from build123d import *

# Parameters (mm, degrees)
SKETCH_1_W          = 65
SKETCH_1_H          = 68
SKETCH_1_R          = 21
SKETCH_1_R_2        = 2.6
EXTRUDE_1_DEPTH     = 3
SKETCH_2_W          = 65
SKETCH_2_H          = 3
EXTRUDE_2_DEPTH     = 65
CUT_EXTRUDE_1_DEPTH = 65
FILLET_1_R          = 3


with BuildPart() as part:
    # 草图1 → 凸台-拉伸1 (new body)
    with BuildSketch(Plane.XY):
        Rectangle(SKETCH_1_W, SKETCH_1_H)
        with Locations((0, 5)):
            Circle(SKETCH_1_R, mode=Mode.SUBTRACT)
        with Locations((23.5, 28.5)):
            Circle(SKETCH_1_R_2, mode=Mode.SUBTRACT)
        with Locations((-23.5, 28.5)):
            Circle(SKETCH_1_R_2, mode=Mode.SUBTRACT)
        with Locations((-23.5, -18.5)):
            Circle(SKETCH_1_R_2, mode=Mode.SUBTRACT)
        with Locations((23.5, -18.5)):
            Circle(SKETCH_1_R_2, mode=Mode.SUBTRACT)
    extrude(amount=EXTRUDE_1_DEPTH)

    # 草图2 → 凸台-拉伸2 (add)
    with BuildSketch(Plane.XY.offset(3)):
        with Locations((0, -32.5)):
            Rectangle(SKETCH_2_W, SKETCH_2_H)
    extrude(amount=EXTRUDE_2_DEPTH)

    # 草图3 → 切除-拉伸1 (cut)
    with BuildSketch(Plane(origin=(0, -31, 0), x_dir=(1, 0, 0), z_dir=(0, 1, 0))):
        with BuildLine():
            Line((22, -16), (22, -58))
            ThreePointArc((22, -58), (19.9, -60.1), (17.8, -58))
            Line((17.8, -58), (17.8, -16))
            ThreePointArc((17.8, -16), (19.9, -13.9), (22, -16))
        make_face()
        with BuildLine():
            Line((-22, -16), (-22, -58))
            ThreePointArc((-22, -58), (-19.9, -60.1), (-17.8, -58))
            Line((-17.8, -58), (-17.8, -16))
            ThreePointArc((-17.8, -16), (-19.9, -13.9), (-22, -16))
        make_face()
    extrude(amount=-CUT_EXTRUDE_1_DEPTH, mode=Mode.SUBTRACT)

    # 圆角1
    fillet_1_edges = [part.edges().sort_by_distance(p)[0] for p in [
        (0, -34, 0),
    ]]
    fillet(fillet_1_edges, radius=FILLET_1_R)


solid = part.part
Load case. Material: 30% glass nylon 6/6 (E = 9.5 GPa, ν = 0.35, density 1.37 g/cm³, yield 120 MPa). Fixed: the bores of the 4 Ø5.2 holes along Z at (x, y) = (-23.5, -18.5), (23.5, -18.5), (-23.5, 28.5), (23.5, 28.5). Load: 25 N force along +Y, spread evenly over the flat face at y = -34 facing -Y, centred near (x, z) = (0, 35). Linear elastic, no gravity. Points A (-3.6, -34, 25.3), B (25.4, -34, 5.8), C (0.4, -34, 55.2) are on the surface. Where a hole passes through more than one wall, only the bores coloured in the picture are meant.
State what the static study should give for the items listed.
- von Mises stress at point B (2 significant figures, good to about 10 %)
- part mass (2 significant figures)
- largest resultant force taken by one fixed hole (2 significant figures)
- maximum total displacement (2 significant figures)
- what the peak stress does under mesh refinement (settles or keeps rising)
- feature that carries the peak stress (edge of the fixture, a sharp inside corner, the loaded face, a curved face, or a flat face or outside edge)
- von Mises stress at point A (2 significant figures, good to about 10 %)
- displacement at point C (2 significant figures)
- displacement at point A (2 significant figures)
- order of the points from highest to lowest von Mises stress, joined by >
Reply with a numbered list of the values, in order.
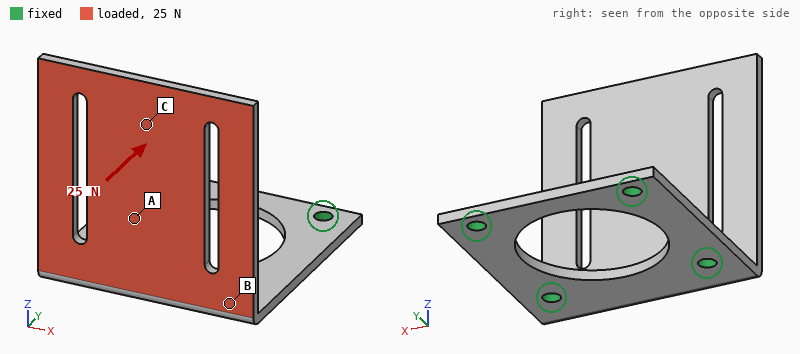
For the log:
1. 6.5 MPa
2. 28 g
3. 14 N
4. 1.2 mm
5. keeps rising
6. edge of the fixture
7. 3.6 MPa
8. 0.96 mm
9. 0.34 mm
10. B > A > C
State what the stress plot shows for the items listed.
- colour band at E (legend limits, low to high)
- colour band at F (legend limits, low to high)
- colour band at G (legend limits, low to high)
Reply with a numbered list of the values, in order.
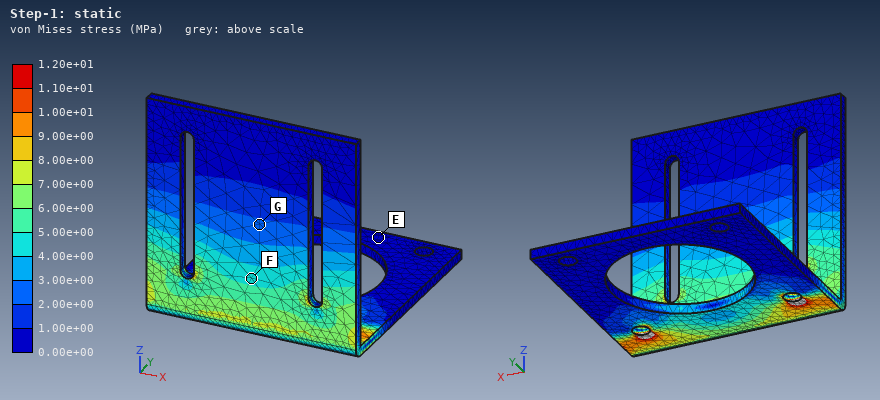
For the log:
1. 0.00e+00 to 1.00e+00 MPa
2. 4.00e+00 to 5.00e+00 MPa
3. 2.00e+00 to 3.00e+00 MPa
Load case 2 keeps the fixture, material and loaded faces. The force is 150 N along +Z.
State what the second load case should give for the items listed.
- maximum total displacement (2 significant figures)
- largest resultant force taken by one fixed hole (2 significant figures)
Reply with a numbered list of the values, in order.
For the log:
1. 1.1 mm
2. 76 N
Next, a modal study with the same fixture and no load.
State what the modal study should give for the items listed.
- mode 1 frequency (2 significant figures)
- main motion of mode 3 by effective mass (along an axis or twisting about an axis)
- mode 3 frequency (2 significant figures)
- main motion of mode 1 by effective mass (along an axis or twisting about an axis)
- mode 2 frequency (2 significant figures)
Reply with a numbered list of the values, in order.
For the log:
1. 220 Hz
2. along X
3. 1000 Hz
4. along Y
5. 610 Hz
